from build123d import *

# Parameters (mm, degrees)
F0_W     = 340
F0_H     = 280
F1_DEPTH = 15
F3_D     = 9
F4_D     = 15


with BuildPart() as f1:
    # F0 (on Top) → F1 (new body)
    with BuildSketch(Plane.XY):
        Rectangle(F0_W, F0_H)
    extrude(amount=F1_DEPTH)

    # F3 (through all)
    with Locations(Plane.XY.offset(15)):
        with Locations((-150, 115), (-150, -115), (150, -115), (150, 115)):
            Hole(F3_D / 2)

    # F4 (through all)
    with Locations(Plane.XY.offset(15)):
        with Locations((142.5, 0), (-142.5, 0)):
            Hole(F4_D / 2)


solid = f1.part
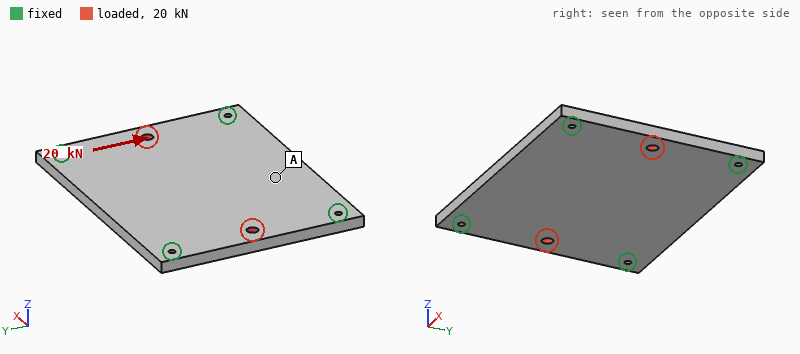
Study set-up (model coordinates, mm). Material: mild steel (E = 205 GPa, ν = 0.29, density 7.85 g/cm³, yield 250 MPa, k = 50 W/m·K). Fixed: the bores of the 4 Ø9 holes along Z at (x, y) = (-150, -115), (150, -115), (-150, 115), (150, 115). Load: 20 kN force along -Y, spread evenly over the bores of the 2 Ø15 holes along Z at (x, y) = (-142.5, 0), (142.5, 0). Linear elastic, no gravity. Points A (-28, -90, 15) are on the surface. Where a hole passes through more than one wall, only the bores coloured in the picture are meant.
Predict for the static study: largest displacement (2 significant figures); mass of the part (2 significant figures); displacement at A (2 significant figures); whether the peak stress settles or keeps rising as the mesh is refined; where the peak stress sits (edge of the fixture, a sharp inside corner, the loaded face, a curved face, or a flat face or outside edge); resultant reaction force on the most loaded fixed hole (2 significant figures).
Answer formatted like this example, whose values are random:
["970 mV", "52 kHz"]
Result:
["4.3 µm", "11 kg", "2.3 µm", "keeps rising", "edge of the fixture", "5.0 kN"]
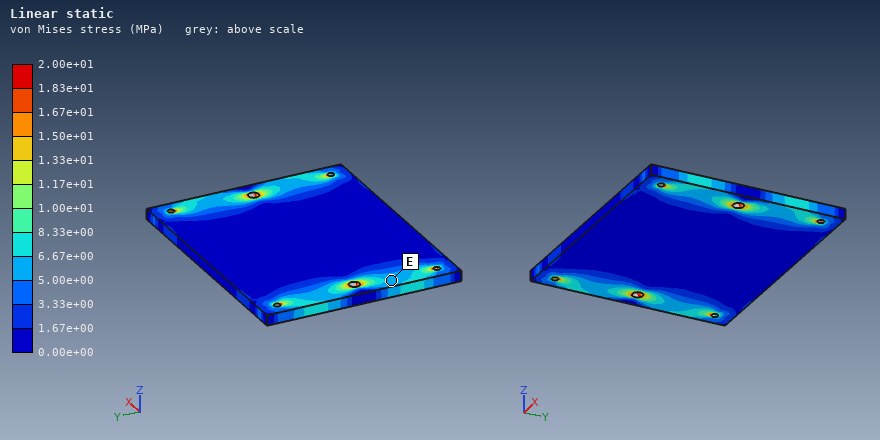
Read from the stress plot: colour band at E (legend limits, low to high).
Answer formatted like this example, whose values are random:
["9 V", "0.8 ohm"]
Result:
["5.00e+00 to 6.67e+00 MPa"]
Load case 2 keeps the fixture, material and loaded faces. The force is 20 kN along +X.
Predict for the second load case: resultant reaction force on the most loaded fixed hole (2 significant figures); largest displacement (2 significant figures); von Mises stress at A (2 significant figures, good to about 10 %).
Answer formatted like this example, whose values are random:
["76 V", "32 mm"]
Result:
["5.4 kN", "7.8 µm", "3.0 MPa"]
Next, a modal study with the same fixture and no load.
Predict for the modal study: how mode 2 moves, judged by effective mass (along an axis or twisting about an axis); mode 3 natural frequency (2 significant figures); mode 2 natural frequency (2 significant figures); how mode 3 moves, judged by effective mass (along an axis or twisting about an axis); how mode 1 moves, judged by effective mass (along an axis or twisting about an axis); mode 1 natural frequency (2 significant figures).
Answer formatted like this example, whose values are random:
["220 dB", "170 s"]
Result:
["twisting about X", "1300 Hz", "990 Hz", "twisting about Y", "along Z", "620 Hz"]
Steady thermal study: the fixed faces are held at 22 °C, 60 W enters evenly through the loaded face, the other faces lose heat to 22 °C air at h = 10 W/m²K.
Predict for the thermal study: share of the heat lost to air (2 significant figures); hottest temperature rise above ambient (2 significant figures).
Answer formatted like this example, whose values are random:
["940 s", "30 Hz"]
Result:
["34 %", "30 K"]
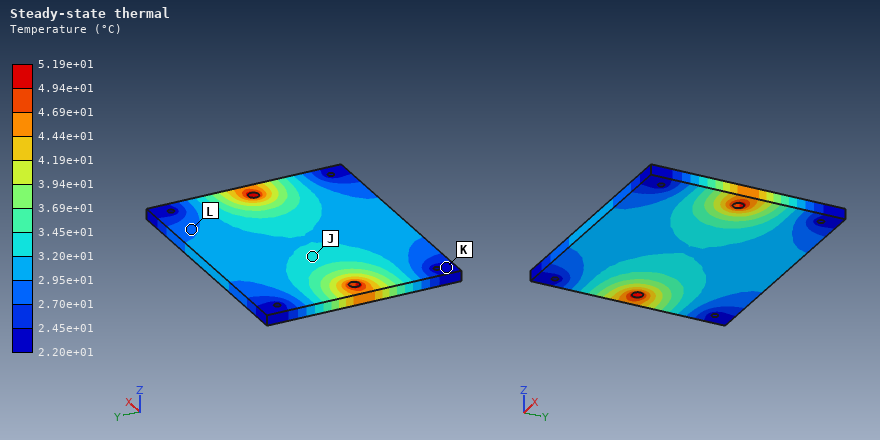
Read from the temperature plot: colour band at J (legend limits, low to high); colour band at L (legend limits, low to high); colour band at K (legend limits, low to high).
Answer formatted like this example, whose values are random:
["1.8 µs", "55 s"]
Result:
["3.20e+01 to 3.45e+01 °C", "2.70e+01 to 2.95e+01 °C", "2.20e+01 to 2.45e+01 °C"]
